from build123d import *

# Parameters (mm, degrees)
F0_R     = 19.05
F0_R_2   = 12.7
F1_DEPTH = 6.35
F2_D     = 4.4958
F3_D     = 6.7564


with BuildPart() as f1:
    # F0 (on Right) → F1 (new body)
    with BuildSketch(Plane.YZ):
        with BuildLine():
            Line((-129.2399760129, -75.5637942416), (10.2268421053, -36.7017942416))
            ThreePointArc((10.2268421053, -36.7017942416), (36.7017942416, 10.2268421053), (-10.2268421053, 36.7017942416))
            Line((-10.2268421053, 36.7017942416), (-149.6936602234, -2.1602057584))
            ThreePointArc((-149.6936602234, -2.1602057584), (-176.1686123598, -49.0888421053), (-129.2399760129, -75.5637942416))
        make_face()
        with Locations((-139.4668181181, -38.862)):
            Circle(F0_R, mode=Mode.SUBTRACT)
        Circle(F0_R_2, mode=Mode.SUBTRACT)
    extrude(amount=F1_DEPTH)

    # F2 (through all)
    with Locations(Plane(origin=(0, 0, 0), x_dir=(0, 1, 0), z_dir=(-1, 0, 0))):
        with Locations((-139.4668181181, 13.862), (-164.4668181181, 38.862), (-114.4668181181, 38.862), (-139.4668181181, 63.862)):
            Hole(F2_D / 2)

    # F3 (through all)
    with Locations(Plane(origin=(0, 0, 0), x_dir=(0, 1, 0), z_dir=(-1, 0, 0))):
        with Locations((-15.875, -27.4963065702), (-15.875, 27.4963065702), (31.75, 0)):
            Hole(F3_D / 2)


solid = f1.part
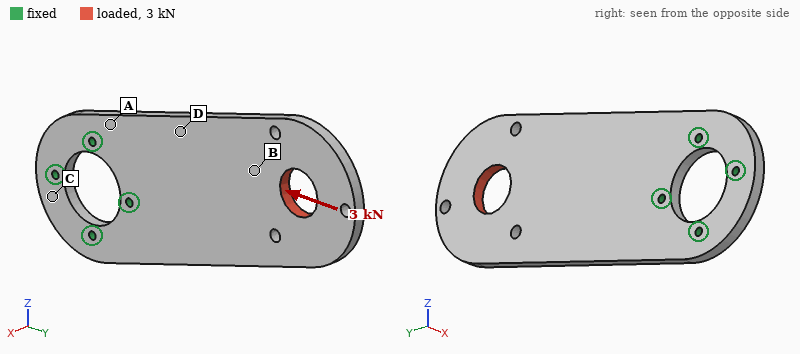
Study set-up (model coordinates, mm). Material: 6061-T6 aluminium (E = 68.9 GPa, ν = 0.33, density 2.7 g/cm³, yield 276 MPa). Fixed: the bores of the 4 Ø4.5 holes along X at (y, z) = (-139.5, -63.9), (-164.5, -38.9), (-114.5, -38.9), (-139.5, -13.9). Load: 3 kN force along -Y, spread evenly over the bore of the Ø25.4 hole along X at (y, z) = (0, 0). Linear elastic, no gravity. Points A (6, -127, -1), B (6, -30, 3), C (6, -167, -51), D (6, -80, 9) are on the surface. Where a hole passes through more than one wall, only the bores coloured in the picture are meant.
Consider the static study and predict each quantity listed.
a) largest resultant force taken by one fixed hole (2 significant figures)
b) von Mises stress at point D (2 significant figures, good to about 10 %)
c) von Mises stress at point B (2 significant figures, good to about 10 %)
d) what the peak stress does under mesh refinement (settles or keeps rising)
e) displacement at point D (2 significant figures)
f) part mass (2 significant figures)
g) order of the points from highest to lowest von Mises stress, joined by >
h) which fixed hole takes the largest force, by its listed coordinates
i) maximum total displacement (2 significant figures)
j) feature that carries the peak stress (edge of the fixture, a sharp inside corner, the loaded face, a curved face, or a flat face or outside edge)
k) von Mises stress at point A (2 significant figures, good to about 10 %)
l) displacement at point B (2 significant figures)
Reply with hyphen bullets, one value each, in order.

- 2.8 kN
- 14 MPa
- 8.4 MPa
- keeps rising
- 27 µm
- 240 g
- A > D > B > C
- (-139.5, -13.9)
- 85 µm
- edge of the fixture
- 20 MPa
- 47 µm
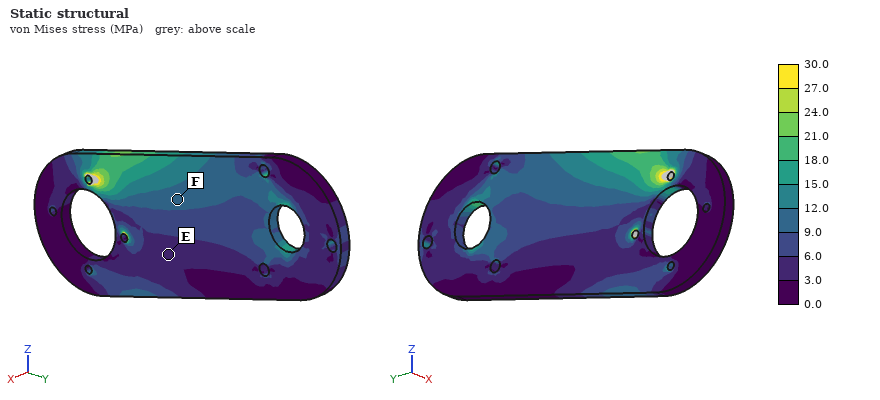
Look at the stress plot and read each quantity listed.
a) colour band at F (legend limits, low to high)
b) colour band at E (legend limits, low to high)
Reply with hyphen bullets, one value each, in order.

- 9.0 to 12.0 MPa
- 3.0 to 6.0 MPa
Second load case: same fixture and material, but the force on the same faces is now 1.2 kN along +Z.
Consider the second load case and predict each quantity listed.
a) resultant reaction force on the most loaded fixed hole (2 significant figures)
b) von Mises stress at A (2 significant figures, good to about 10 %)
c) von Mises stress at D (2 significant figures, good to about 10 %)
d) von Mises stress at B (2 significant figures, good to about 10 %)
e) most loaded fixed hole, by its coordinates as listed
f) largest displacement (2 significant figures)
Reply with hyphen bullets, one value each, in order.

- 2.5 kN
- 19 MPa
- 11 MPa
- 5.9 MPa
- (-139.5, -13.9)
- 0.12 mm
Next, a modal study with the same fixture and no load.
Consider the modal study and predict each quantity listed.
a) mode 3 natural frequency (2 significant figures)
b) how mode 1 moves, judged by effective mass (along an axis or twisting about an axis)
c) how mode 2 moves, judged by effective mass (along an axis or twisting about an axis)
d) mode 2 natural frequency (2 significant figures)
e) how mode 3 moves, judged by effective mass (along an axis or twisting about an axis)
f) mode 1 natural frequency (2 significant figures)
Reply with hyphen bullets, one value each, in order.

- 1200 Hz
- along X
- twisting about Y
- 880 Hz
- along X
- 230 Hz
